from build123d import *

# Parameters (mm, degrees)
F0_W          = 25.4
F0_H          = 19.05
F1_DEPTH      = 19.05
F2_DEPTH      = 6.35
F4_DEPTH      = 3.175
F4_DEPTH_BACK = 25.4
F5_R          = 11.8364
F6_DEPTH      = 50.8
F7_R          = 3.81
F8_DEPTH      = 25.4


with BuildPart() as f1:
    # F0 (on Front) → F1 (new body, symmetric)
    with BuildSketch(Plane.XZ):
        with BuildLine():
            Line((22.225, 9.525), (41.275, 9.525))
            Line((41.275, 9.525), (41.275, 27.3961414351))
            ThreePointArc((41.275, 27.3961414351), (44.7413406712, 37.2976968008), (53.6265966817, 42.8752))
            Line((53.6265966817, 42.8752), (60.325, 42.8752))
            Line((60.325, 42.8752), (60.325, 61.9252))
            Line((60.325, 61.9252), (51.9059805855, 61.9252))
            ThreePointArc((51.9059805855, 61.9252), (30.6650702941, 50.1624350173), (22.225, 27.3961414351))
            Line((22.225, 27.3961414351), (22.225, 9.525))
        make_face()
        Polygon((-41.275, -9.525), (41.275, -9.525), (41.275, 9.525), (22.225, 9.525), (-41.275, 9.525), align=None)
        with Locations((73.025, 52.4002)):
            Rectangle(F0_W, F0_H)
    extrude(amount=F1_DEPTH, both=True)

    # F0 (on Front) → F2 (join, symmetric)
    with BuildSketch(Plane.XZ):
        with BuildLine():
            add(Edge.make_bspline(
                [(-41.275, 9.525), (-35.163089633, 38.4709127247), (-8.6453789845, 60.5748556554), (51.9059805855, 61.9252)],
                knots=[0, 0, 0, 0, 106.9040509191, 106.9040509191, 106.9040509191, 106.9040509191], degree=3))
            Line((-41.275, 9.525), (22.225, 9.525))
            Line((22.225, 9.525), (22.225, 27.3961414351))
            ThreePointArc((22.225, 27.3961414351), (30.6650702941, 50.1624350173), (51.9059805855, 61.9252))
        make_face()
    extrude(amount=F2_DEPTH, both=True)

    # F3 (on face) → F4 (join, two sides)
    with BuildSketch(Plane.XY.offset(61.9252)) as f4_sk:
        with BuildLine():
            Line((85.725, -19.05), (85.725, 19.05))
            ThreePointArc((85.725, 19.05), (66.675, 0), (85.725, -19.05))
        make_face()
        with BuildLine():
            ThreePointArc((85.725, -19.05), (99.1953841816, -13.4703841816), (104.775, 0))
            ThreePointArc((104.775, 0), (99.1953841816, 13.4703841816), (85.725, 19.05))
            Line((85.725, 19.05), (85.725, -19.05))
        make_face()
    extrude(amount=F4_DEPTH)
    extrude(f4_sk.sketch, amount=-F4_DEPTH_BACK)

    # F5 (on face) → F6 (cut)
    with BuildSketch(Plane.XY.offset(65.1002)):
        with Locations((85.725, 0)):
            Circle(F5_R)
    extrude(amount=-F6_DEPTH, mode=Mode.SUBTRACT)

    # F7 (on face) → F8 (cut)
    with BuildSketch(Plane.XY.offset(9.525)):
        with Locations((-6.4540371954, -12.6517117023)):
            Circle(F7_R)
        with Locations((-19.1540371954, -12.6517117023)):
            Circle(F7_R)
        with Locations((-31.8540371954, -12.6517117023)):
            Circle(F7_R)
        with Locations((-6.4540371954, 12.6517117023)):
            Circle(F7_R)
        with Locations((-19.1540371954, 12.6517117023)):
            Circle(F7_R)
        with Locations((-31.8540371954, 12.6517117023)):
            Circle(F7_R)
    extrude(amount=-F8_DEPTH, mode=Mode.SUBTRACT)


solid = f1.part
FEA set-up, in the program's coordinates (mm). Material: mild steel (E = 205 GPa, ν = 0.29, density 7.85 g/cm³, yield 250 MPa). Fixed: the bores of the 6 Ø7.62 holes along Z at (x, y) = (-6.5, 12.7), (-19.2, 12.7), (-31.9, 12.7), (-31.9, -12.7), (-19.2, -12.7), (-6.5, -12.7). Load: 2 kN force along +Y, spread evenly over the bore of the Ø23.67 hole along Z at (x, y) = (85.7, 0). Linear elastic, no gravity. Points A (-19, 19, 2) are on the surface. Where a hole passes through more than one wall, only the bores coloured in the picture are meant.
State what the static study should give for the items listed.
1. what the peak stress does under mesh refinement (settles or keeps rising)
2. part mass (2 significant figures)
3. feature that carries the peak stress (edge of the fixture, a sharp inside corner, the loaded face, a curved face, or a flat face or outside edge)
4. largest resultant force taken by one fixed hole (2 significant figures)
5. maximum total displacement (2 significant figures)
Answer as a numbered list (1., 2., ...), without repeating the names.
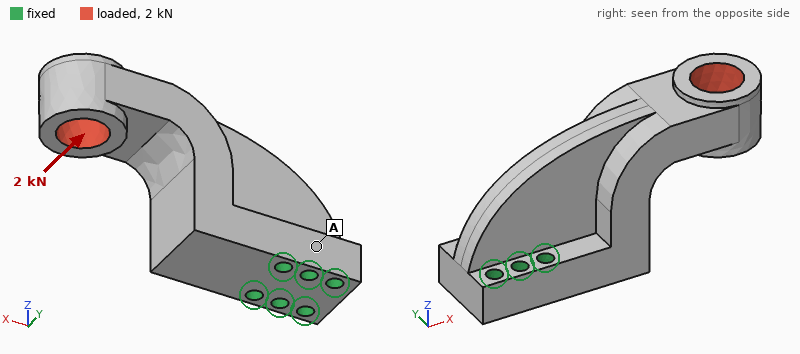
1. keeps rising
2. 1.2 kg
3. edge of the fixture
4. 6.8 kN
5. 0.10 mm
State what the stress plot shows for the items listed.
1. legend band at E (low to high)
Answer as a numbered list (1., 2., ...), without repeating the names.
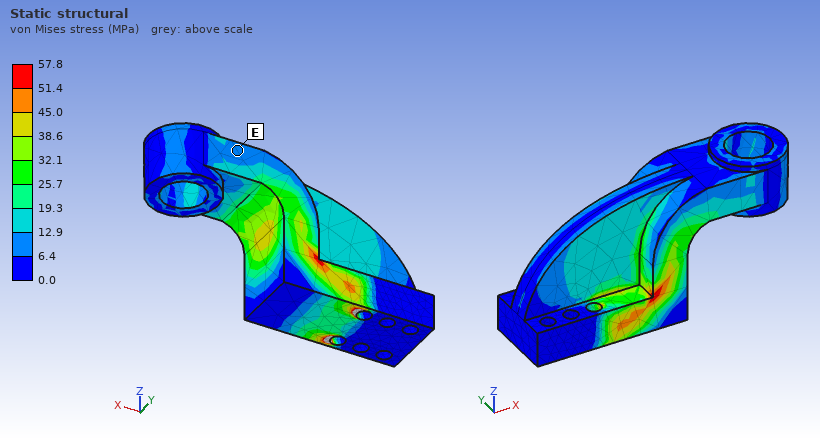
1. 6.4 to 12.9 MPa
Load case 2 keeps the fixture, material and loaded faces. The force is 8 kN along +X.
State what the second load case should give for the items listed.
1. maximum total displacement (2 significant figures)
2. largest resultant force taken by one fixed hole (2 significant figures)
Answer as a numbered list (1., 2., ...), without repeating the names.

1. 62 µm
2. 4.6 kN
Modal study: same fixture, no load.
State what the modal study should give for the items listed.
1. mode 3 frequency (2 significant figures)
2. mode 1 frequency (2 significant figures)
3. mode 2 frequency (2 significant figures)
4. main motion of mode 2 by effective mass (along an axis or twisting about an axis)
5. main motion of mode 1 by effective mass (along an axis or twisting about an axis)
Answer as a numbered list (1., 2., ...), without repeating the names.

1. 3900 Hz
2. 1500 Hz
3. 2100 Hz
4. along Z
5. along Y
